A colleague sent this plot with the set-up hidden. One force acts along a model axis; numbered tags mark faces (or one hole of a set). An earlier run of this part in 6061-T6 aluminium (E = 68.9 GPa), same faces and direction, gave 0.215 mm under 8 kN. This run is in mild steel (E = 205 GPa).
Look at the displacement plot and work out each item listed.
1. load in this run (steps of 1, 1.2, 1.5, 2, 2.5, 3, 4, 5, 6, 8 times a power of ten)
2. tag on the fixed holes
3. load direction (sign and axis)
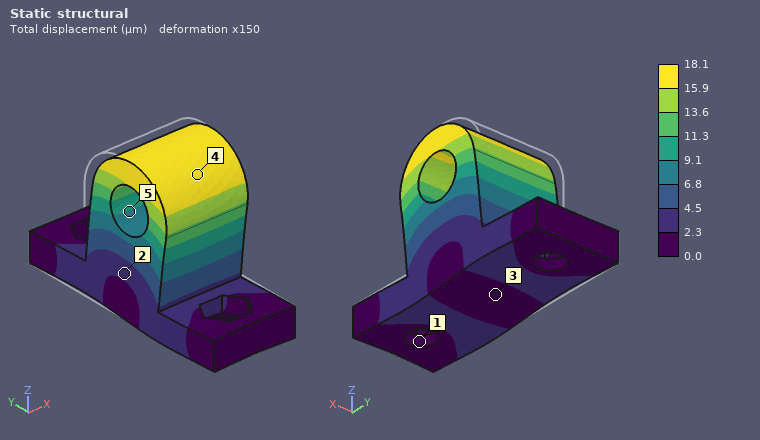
2 kN
1
-Y
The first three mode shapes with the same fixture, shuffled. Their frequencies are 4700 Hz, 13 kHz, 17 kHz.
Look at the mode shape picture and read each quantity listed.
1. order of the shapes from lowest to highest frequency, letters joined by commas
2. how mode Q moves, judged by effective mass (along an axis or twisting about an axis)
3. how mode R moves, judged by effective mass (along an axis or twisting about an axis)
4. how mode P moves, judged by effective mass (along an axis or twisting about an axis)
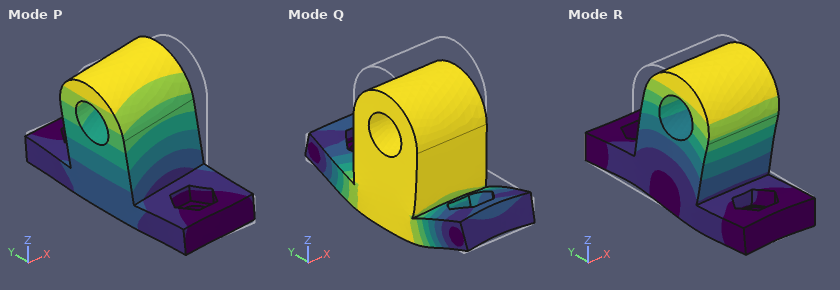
P, R, Q
along Z
along Y
along X
